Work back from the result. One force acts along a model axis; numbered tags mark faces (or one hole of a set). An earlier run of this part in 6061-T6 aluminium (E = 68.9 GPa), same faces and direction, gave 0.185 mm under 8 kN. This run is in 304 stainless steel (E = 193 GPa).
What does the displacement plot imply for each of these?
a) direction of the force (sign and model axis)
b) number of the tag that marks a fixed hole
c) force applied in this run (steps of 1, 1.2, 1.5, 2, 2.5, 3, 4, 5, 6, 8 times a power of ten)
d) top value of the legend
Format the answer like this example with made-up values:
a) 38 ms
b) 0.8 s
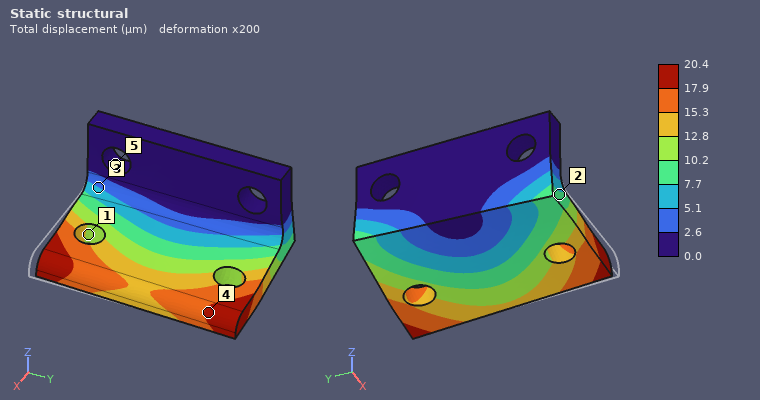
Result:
a) +Y
b) 5
c) 2.5 kN
d) 20.4 µm
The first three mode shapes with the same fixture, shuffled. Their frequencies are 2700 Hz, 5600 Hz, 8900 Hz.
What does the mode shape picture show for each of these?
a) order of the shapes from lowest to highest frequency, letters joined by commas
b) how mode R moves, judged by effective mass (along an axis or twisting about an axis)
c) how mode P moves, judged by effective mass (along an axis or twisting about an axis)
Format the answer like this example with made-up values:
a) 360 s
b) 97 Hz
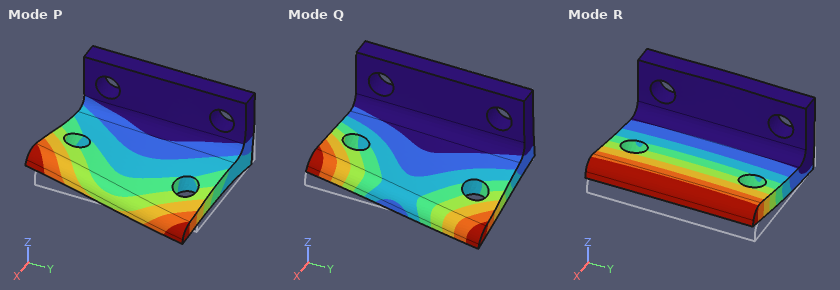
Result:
a) R, Q, P
b) along Z
c) along Y
